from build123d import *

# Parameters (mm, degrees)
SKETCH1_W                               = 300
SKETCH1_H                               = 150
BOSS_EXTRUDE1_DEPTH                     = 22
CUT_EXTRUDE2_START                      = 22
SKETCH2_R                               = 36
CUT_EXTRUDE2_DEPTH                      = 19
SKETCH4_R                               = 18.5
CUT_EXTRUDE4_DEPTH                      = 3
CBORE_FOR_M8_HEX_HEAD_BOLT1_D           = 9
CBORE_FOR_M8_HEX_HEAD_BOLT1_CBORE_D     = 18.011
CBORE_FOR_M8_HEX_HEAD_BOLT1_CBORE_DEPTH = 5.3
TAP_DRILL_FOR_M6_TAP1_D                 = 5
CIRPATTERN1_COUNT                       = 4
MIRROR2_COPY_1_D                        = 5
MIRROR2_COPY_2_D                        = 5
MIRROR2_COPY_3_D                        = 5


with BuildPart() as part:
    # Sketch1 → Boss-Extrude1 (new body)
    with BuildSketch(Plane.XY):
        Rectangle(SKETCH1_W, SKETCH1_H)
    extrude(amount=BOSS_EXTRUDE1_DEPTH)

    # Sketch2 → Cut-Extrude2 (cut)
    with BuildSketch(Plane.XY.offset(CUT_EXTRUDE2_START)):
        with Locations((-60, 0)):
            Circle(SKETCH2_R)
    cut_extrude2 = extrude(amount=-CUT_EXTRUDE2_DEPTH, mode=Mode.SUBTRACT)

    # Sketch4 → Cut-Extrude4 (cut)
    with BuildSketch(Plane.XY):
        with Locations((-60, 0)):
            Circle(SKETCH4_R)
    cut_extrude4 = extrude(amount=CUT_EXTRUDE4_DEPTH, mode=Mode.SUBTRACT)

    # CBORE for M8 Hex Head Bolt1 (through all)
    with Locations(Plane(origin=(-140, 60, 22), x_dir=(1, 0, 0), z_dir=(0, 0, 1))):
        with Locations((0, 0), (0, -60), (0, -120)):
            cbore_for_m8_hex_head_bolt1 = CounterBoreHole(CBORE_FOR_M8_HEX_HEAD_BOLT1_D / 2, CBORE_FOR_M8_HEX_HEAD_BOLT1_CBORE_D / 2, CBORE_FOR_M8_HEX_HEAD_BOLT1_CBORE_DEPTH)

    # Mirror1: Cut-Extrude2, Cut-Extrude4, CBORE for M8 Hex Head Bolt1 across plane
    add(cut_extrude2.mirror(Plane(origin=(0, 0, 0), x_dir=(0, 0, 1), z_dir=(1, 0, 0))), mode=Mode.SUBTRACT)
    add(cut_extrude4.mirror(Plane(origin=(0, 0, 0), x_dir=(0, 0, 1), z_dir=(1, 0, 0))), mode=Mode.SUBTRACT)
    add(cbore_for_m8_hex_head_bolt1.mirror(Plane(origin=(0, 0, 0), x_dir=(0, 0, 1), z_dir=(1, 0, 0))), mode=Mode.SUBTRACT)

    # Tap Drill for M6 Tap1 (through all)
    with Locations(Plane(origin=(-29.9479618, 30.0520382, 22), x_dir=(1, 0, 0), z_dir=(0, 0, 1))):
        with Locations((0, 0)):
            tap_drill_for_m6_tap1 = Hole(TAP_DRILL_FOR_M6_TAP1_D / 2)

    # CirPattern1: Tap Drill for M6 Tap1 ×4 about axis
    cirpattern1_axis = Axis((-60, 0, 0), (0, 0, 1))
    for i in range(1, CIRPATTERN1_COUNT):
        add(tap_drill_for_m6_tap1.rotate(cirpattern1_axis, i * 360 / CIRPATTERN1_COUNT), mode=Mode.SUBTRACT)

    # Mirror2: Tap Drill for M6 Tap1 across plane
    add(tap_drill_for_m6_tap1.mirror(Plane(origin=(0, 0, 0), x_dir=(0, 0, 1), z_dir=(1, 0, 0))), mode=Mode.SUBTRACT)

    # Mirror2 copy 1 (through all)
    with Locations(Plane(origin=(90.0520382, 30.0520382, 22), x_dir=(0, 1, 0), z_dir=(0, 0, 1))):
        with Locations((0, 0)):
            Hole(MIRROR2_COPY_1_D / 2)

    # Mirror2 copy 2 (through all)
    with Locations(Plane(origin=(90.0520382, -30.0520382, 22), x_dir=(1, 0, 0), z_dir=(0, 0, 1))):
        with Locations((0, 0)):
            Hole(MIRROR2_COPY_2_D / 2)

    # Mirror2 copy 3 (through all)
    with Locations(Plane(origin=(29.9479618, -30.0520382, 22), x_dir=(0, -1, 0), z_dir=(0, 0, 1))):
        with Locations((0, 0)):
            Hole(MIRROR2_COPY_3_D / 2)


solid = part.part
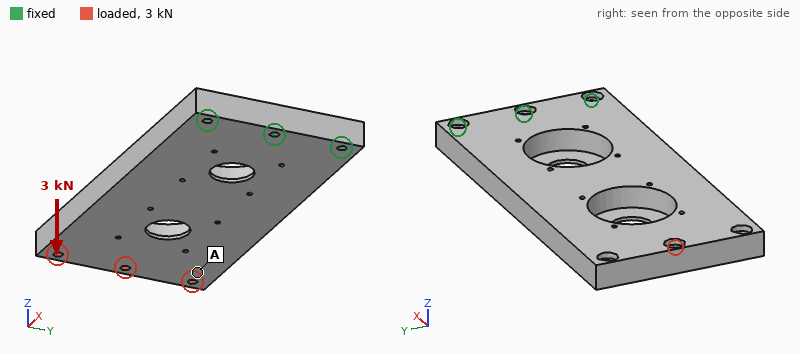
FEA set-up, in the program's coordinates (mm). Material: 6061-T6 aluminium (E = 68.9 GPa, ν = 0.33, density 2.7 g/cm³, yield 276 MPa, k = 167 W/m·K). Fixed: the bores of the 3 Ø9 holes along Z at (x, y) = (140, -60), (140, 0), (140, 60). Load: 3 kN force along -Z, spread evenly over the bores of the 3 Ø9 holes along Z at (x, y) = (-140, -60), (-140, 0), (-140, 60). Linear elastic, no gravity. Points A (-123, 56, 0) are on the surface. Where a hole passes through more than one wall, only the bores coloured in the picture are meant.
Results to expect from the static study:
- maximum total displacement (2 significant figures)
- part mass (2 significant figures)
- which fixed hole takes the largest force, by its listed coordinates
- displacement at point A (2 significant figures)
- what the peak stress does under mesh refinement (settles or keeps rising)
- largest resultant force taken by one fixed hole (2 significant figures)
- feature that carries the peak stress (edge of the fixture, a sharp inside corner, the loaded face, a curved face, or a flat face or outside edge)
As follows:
3.9 mm
2.2 kg
(140, 0)
3.3 mm
keeps rising
3.8 kN
edge of the fixture
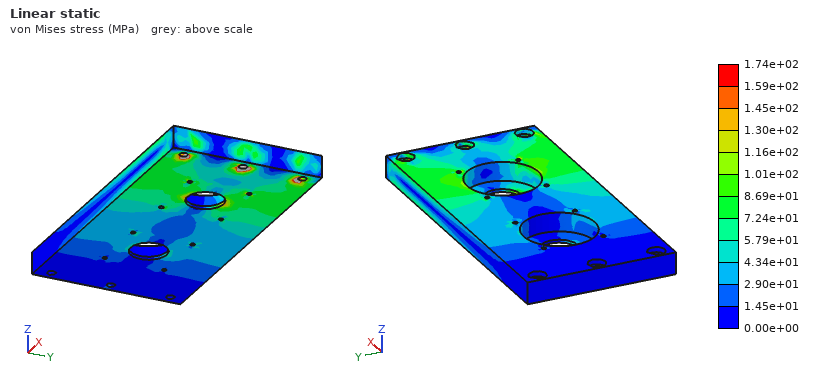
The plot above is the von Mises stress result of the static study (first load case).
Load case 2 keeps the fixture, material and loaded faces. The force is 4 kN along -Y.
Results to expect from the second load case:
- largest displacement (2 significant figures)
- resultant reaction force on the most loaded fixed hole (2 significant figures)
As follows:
0.13 mm
9.2 kN
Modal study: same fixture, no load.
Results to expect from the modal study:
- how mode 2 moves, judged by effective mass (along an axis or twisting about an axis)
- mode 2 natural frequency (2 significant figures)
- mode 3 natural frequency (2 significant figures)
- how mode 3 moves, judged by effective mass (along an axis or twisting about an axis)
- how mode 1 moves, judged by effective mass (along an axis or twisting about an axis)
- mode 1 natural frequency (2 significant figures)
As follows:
twisting about X
720 Hz
1100 Hz
along Y
along Z
180 Hz
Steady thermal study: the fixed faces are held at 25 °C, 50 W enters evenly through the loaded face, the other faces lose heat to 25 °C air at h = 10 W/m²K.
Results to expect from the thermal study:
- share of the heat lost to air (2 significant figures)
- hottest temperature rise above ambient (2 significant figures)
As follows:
32 %
30 K
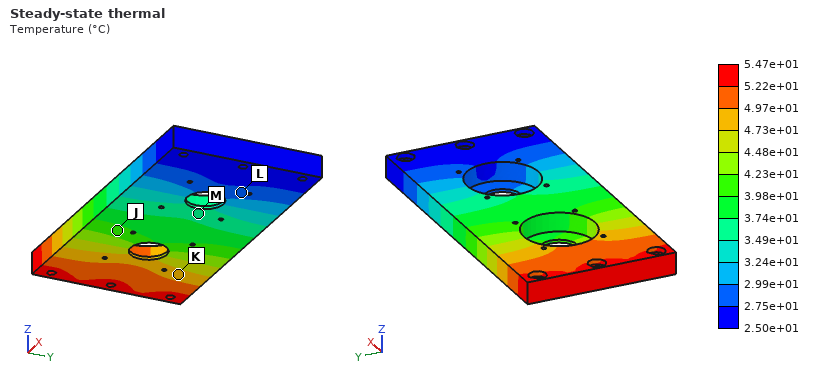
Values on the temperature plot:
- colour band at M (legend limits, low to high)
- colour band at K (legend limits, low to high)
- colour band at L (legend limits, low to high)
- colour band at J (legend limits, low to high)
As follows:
3.49e+01 to 3.74e+01 °C
4.73e+01 to 4.97e+01 °C
2.75e+01 to 2.99e+01 °C
3.98e+01 to 4.23e+01 °C
